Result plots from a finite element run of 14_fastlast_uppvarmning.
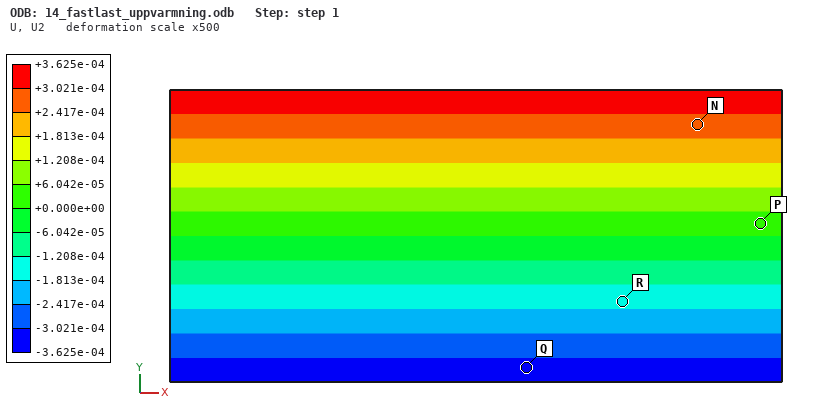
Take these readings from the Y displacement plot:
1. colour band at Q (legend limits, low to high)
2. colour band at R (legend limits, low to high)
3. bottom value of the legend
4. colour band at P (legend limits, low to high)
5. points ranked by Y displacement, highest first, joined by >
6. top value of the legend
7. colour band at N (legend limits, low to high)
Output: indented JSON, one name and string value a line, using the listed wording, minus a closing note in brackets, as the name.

{
  "colour band at Q": "-3.625e-04 to -3.021e-04",
  "colour band at R": "-1.813e-04 to -1.208e-04",
  "bottom value of the legend": "-3.625e-04",
  "colour band at P": "+0.000e+00 to +6.042e-05",
  "points ranked by Y displacement, highest first, joined by >": "N > P > R > Q",
  "top value of the legend": "+3.625e-04",
  "colour band at N": "+2.417e-04 to +3.021e-04"
}
